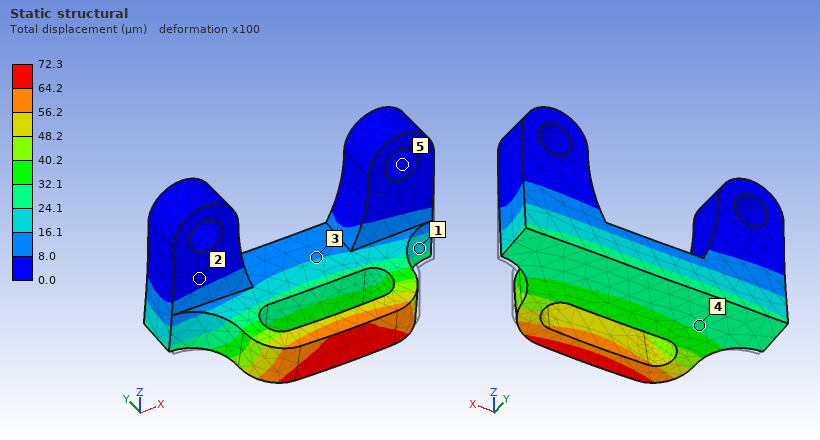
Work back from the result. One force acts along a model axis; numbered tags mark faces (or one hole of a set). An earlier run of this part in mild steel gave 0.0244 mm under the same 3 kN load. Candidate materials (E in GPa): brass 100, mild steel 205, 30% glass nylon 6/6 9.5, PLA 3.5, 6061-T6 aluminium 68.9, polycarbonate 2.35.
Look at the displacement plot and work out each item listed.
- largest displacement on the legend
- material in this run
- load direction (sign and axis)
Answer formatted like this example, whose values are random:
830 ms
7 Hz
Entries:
72.3 µm
6061-T6 aluminium
-Z
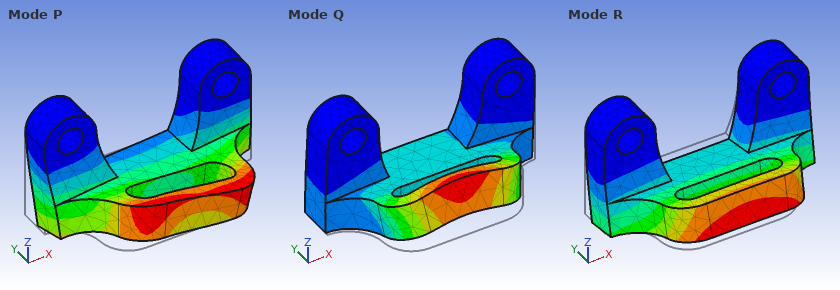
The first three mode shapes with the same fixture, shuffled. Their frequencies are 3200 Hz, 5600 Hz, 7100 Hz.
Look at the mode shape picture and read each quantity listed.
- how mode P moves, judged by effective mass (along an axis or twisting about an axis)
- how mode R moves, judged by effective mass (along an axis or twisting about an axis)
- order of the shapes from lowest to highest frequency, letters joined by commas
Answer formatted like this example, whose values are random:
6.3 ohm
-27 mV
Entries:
along X
along Y
R, P, Q
